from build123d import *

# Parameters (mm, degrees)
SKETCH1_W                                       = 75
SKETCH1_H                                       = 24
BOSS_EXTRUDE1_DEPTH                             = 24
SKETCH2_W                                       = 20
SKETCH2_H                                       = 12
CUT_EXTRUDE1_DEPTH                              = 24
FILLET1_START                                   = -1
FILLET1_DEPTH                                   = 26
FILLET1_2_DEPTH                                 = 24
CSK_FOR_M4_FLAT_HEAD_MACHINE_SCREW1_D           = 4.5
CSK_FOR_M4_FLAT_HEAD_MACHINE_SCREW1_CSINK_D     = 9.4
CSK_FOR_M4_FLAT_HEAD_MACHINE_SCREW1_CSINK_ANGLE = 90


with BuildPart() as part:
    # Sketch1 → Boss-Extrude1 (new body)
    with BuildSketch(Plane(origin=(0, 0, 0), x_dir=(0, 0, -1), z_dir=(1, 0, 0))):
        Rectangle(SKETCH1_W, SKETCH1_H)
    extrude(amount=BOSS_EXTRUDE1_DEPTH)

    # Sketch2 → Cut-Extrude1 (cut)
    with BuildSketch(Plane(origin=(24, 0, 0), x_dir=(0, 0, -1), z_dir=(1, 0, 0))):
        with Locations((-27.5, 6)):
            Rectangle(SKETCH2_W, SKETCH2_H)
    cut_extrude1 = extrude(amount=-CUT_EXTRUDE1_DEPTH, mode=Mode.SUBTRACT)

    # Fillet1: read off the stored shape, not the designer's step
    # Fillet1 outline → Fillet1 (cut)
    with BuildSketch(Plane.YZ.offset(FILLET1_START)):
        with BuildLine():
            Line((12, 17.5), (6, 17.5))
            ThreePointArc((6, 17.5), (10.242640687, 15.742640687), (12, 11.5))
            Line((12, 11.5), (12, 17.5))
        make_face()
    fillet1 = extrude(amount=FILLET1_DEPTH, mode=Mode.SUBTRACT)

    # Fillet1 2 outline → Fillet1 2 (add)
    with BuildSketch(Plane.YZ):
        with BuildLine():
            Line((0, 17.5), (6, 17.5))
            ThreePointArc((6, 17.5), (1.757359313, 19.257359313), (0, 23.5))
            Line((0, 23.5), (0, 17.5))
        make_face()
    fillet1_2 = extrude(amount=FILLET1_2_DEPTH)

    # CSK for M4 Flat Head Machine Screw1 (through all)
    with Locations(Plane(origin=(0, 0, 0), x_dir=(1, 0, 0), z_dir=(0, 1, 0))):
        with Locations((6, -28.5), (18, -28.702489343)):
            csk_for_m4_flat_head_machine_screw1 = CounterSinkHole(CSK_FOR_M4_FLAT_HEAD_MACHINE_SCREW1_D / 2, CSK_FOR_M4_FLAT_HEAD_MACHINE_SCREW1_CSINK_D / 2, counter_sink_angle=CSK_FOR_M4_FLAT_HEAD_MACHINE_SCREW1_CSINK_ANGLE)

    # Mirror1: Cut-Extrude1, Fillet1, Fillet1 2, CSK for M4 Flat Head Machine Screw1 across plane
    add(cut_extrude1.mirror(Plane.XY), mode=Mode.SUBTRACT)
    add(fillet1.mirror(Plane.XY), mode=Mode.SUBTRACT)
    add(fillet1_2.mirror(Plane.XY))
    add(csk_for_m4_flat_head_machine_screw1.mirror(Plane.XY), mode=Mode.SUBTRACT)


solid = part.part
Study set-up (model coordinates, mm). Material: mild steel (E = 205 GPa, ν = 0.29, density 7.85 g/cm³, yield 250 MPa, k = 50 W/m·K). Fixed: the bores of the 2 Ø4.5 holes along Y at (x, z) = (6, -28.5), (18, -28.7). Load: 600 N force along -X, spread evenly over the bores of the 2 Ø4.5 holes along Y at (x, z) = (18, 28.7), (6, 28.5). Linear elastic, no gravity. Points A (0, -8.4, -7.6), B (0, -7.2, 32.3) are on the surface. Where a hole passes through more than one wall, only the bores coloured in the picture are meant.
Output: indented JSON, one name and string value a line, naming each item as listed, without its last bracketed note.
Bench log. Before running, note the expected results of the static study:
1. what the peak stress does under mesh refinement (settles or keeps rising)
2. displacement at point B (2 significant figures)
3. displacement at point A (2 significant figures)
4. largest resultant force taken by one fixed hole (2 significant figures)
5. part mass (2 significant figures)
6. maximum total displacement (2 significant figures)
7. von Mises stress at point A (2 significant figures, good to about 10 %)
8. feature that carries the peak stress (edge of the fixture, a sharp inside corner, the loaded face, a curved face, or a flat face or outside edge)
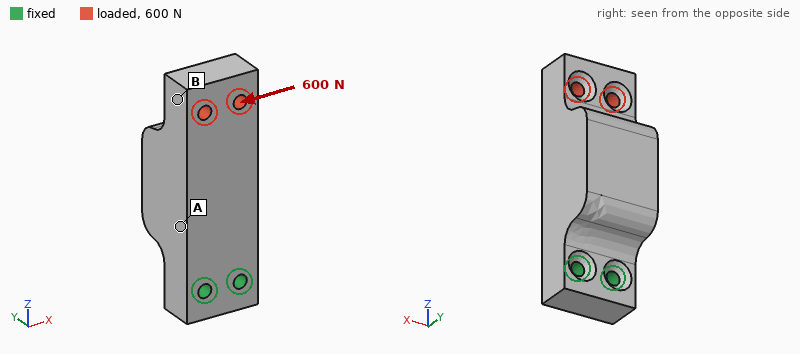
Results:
{
  "what the peak stress does under mesh refinement": "keeps rising",
  "displacement at point B": "16 µm",
  "displacement at point A": "4.4 µm",
  "largest resultant force taken by one fixed hole": "2.3 kN",
  "part mass": "240 g",
  "maximum total displacement": "18 µm",
  "von Mises stress at point A": "14 MPa",
  "feature that carries the peak stress": "edge of the fixture"
}
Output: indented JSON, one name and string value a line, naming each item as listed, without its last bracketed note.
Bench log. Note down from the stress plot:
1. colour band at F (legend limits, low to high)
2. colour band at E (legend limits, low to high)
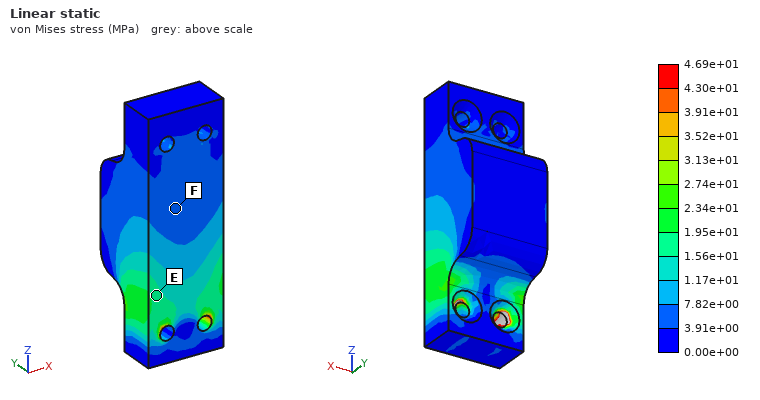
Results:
{
  "colour band at F": "3.91e+00 to 7.82e+00 MPa",
  "colour band at E": "1.56e+01 to 1.95e+01 MPa"
}
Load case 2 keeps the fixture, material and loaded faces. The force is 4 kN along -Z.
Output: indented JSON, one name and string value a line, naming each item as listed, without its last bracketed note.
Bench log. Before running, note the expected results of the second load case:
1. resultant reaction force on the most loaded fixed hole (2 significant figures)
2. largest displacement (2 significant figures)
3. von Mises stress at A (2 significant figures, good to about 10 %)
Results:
{
  "resultant reaction force on the most loaded fixed hole": "2.0 kN",
  "largest displacement": "14 µm",
  "von Mises stress at A": "16 MPa"
}
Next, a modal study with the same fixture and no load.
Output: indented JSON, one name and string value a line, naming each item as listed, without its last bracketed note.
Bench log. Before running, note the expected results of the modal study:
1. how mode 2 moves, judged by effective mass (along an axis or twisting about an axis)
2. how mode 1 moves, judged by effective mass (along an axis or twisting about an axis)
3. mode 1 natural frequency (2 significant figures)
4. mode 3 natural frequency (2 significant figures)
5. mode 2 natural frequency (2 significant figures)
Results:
{
  "how mode 2 moves, judged by effective mass": "along X",
  "how mode 1 moves, judged by effective mass": "along Y",
  "mode 1 natural frequency": "2200 Hz",
  "mode 3 natural frequency": "8600 Hz",
  "mode 2 natural frequency": "3900 Hz"
}
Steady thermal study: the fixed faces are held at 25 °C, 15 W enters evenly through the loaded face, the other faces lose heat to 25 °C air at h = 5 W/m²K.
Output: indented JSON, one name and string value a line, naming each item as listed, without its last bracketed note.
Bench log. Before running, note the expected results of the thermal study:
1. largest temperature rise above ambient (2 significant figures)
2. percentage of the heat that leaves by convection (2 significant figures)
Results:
{
  "largest temperature rise above ambient": "47 K",
  "percentage of the heat that leaves by convection": "5.1 %"
}
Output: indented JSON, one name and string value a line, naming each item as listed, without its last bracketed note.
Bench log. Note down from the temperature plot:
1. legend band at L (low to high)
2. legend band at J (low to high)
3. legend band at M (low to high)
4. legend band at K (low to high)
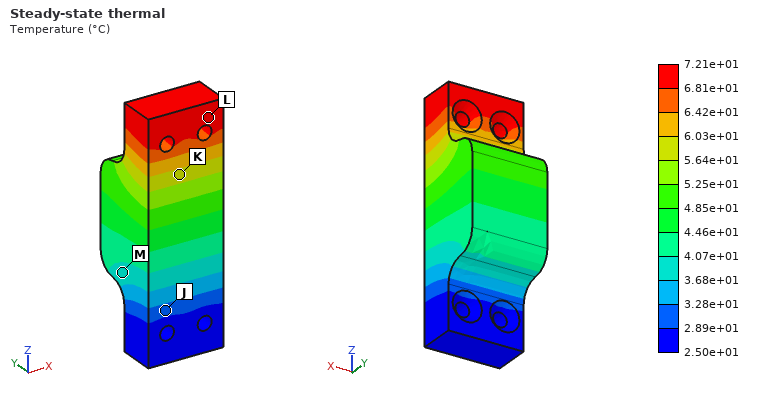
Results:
{
  "legend band at L": "6.81e+01 to 7.21e+01 °C",
  "legend band at J": "2.89e+01 to 3.28e+01 °C",
  "legend band at M": "3.68e+01 to 4.07e+01 °C",
  "legend band at K": "5.64e+01 to 6.03e+01 °C"
}
